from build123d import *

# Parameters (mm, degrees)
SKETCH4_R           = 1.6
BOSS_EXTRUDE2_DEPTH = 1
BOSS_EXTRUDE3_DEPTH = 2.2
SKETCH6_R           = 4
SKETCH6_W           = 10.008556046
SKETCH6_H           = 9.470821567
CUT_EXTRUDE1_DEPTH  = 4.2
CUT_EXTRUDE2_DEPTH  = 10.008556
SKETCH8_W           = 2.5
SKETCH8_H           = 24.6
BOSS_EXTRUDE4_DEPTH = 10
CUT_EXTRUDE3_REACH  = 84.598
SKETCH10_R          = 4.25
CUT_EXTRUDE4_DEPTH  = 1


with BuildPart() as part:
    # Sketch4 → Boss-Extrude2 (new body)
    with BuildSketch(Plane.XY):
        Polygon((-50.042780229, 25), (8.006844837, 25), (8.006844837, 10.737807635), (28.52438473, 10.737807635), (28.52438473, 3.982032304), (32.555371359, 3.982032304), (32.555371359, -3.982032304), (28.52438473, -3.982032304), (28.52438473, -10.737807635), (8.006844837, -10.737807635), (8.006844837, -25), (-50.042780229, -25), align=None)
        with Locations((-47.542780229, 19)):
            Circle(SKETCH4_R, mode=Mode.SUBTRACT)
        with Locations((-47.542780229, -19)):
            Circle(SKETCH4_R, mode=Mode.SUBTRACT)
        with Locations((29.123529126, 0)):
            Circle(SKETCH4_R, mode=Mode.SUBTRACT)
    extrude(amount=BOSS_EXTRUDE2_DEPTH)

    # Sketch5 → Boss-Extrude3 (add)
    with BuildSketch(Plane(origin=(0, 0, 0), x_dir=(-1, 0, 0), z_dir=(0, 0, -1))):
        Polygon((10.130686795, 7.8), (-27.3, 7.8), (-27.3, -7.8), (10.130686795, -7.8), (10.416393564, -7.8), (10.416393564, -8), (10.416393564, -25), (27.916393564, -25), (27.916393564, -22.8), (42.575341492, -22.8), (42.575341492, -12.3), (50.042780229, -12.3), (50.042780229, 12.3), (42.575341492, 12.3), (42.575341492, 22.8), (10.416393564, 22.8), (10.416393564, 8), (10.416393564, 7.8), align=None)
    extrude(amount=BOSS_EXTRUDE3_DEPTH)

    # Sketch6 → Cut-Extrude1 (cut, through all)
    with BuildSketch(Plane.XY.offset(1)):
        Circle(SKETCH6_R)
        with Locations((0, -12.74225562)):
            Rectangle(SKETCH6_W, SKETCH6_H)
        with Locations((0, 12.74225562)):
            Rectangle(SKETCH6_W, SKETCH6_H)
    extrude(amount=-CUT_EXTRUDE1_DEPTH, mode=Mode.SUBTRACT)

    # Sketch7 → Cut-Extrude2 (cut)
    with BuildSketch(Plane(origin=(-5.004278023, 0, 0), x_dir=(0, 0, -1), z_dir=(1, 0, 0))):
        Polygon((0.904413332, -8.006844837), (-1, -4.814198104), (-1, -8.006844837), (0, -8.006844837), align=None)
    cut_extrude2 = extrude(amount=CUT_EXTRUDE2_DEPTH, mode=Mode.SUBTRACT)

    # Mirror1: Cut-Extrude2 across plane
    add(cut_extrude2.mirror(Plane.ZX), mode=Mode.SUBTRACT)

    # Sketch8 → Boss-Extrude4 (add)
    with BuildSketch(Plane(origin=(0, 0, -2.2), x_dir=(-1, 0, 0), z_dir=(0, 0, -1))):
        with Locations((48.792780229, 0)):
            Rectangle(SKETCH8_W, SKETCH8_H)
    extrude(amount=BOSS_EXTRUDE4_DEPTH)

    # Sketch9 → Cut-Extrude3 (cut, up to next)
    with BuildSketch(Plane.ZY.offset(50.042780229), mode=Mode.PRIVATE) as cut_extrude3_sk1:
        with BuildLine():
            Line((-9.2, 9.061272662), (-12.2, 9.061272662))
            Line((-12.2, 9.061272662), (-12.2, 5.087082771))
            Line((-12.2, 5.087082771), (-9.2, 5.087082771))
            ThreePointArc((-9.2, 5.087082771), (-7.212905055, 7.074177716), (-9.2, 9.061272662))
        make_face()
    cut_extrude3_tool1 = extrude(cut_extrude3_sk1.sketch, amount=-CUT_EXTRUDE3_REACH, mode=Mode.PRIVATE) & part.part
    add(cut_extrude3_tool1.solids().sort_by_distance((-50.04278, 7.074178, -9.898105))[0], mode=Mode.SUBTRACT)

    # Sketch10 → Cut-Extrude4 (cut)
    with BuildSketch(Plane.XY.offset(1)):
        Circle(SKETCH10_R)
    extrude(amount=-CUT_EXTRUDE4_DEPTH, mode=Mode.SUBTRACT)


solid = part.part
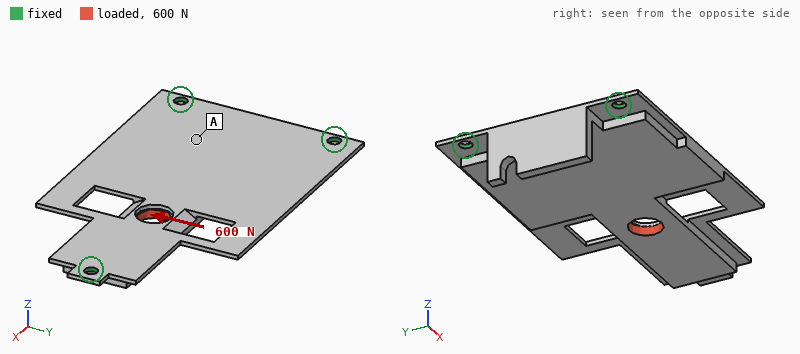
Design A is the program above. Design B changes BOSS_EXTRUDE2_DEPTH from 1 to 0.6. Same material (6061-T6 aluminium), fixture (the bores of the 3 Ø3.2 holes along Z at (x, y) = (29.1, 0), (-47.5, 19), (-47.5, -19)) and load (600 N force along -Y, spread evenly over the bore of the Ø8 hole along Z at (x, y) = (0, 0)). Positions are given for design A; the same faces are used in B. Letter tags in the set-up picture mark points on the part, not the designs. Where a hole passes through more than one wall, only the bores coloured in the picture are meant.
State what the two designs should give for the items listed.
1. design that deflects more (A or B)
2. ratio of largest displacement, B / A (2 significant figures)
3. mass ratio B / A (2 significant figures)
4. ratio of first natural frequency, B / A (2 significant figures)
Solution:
B
1.3
0.86
0.85
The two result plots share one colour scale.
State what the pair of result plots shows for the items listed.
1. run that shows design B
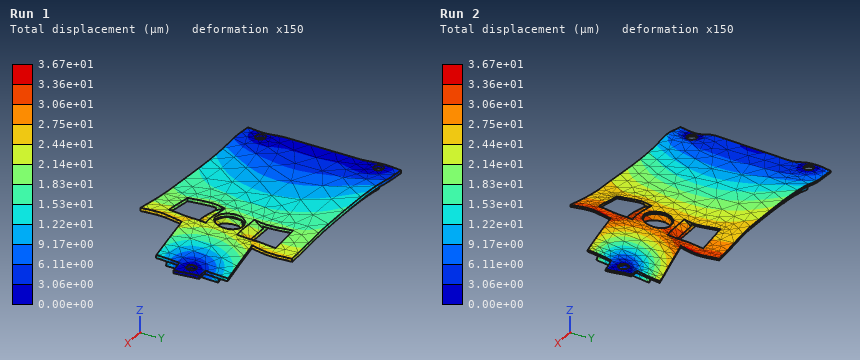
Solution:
Run 2
